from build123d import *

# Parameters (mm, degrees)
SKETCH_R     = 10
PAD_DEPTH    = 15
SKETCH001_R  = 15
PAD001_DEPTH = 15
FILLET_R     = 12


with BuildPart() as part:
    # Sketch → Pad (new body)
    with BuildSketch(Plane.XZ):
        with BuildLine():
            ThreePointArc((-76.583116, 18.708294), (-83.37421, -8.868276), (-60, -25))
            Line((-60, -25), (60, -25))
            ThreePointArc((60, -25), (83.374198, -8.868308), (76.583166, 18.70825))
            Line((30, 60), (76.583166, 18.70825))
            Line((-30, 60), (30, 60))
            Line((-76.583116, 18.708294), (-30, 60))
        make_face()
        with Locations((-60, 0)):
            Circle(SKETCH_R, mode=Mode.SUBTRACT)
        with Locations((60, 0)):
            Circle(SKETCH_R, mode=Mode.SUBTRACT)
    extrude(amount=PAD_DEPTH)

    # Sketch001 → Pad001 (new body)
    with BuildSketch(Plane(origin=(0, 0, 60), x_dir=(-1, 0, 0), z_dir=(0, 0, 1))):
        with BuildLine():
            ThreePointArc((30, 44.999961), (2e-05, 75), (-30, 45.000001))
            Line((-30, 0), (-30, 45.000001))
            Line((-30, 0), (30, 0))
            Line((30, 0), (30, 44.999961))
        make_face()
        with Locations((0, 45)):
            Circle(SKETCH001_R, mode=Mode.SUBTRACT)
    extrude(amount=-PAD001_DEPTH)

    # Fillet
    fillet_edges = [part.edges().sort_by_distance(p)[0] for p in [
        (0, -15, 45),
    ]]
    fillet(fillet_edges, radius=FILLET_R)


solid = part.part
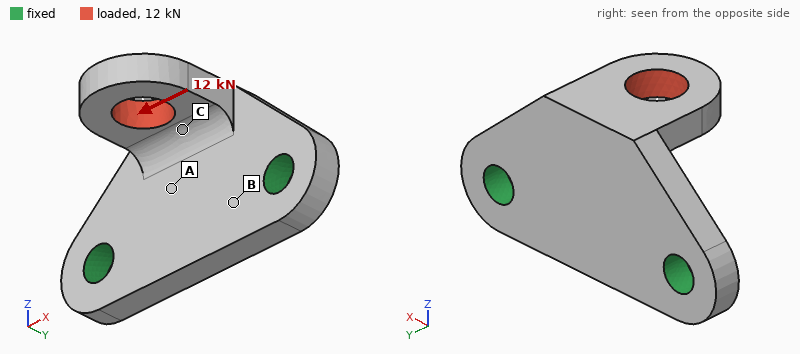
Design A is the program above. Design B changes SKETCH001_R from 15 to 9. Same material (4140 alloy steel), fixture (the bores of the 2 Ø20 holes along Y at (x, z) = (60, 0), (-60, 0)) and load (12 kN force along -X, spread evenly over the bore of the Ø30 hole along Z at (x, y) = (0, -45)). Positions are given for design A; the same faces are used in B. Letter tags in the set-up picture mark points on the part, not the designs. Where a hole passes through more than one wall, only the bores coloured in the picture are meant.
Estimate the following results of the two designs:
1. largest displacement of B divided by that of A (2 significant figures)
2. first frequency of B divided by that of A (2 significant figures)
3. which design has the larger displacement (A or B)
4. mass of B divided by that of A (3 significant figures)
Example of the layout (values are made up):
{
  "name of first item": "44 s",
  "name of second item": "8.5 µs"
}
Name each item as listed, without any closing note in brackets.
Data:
{
  "largest displacement of B divided by that of A": "0.89",
  "first frequency of B divided by that of A": "0.95",
  "which design has the larger displacement": "A",
  "mass of B divided by that of A": "1.03"
}
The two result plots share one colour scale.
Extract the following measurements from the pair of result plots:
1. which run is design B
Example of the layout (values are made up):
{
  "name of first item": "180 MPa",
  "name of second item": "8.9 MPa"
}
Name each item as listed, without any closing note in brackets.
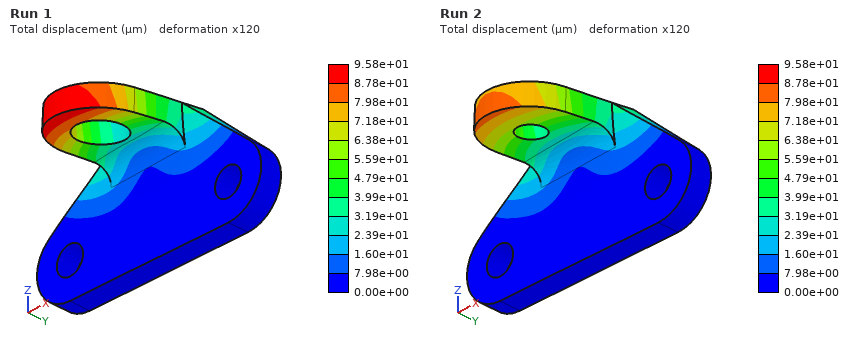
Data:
{
  "which run is design B": "Run 2"
}
